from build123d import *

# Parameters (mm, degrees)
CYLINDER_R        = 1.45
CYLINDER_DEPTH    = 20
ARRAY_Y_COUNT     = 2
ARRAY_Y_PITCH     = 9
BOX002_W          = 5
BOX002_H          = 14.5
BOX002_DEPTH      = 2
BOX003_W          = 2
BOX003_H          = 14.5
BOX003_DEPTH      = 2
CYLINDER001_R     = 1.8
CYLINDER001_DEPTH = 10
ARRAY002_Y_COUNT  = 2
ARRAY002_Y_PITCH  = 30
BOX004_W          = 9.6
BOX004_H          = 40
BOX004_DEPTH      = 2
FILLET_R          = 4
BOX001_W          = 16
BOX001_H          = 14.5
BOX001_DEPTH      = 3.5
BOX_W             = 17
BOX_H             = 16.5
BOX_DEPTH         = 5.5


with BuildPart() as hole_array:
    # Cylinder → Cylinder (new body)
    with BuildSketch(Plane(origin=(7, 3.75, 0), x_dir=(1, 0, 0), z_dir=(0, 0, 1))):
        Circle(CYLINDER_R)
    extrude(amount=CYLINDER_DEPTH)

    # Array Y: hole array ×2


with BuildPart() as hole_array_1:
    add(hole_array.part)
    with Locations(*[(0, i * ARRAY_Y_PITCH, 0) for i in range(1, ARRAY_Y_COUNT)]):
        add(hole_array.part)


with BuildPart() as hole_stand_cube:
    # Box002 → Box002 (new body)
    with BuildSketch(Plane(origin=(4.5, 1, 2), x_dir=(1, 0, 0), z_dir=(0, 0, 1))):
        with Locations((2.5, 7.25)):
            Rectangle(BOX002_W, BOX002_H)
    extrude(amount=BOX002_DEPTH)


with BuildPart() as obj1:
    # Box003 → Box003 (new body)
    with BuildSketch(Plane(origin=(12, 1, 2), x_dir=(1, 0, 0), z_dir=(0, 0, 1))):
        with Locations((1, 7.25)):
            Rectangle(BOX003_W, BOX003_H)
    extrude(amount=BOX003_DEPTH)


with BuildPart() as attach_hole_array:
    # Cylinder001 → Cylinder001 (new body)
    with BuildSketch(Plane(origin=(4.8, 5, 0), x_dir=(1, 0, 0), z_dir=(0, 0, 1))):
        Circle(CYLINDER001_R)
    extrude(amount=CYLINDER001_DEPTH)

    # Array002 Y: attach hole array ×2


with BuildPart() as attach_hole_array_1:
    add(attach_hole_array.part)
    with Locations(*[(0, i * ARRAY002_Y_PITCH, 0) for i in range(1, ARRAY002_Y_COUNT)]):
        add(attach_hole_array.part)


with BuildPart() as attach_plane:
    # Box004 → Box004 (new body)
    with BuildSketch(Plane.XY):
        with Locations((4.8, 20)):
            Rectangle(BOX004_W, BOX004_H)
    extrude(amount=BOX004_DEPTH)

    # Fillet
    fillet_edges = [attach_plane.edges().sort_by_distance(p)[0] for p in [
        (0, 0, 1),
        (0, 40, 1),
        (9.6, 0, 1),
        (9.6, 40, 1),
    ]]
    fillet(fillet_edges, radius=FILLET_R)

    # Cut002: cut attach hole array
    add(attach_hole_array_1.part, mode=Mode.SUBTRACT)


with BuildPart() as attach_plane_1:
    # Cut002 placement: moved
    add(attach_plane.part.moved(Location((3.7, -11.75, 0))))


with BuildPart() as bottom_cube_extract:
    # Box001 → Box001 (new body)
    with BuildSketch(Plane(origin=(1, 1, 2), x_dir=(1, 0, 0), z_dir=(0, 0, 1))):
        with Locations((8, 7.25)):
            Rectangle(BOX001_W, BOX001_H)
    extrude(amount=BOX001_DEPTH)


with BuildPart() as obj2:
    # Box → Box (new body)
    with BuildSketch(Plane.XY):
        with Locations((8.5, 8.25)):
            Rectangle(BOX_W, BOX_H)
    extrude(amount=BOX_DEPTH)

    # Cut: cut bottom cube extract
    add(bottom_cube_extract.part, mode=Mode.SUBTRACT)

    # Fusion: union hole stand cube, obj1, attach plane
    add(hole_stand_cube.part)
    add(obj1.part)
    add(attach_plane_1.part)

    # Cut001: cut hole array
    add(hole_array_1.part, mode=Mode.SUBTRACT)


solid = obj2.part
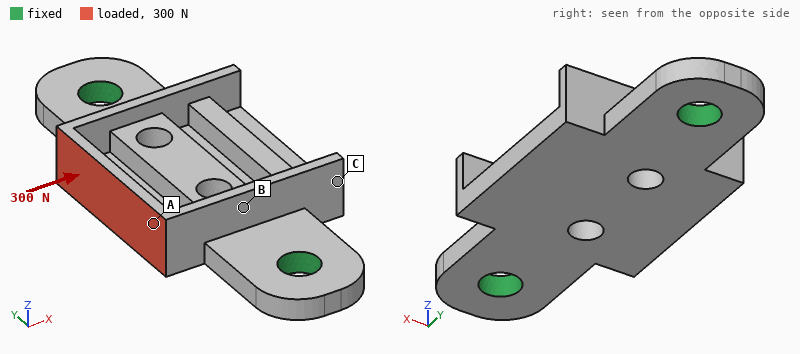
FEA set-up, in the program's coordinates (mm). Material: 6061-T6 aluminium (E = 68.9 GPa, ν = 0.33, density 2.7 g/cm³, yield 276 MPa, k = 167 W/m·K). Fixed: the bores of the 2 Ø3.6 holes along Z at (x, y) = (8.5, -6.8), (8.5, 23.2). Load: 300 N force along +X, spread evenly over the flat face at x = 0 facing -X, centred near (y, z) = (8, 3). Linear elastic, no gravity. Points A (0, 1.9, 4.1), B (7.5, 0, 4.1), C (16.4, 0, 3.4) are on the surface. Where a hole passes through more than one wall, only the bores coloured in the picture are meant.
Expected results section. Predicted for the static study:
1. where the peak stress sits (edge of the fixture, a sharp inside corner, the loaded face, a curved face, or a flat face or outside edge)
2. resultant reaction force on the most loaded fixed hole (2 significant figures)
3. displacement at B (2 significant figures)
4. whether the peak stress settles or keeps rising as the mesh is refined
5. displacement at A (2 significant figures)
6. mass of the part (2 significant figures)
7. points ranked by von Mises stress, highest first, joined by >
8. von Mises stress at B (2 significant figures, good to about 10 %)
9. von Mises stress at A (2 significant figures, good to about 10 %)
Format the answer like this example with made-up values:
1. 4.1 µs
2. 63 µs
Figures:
1. edge of the fixture
2. 150 N
3. 10 µm
4. keeps rising
5. 26 µm
6. 3.4 g
7. A > B > C
8. 17 MPa
9. 49 MPa
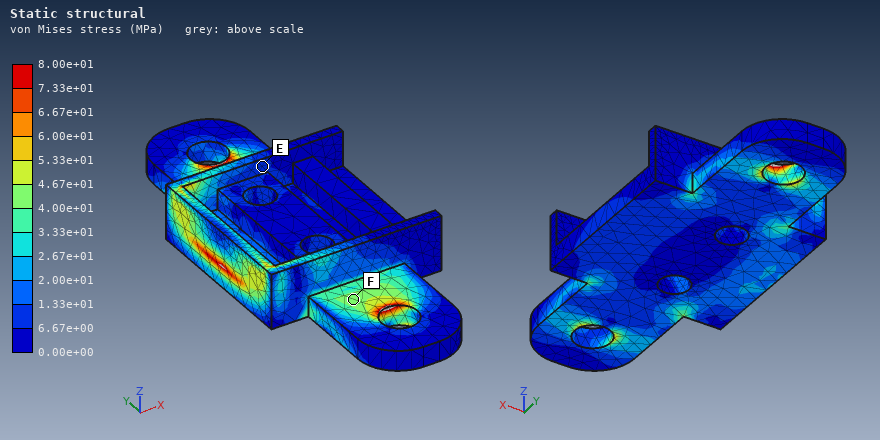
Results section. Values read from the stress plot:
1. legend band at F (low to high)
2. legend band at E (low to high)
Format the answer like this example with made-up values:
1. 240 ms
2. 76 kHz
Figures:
1. 4.00e+01 to 4.67e+01 MPa
2. 6.67e+00 to 1.33e+01 MPa
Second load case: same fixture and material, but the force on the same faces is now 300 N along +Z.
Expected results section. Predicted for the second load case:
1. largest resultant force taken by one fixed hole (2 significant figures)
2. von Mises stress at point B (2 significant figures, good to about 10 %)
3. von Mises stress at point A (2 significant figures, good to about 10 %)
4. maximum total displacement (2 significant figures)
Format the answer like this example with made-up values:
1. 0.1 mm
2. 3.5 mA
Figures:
1. 190 N
2. 46 MPa
3. 54 MPa
4. 0.13 mm
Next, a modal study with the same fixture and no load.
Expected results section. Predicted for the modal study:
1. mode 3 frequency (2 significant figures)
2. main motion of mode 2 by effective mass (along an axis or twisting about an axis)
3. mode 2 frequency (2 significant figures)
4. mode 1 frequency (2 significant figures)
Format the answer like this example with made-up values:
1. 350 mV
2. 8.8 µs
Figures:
1. 27 kHz
2. along Z
3. 13 kHz
4. 9800 Hz
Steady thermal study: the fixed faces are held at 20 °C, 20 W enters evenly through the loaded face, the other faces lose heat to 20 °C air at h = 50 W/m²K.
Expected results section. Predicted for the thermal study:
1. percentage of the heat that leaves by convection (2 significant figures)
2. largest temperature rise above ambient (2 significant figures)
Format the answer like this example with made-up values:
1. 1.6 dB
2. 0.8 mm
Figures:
1. 7.1 %
2. 49 K
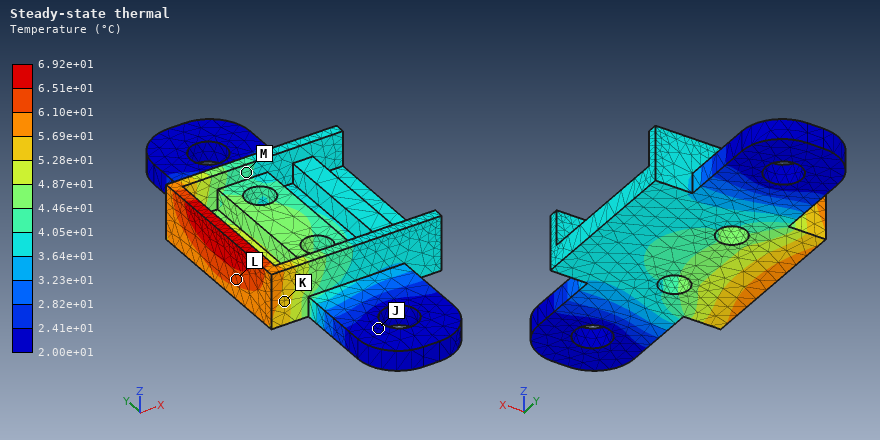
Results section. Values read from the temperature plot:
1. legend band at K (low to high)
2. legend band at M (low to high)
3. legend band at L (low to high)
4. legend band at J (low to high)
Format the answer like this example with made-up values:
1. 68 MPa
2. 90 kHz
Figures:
1. 5.28e+01 to 5.69e+01 °C
2. 4.05e+01 to 4.46e+01 °C
3. 6.10e+01 to 6.51e+01 °C
4. 2.00e+01 to 2.41e+01 °C
